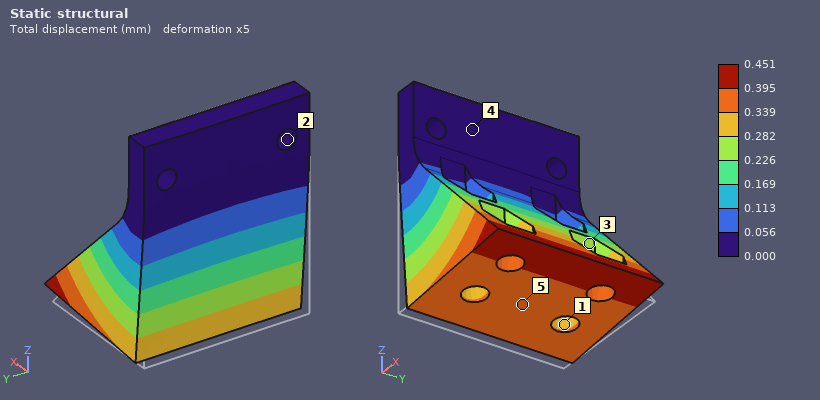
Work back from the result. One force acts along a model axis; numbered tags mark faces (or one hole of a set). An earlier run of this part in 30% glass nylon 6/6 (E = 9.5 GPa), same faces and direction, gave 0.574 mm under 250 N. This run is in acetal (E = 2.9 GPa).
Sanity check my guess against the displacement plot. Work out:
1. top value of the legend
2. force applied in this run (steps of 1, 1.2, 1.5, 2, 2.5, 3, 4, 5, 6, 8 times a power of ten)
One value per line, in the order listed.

0.451 mm
60 N
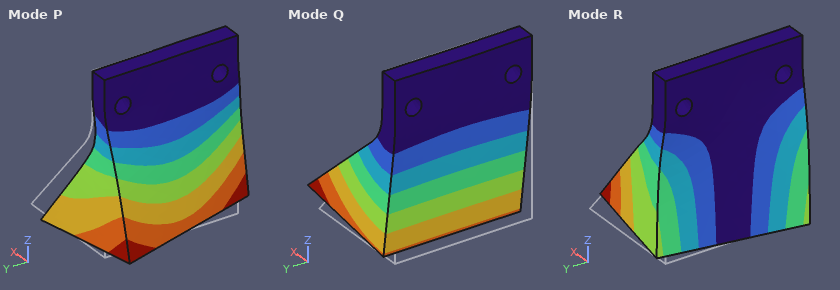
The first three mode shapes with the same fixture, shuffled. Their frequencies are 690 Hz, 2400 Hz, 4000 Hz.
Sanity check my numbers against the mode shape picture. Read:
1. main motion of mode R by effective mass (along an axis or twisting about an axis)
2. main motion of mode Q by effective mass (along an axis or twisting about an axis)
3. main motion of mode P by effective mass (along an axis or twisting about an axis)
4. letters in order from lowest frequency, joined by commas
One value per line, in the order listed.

along Y
along X
along Y
Q, R, P
